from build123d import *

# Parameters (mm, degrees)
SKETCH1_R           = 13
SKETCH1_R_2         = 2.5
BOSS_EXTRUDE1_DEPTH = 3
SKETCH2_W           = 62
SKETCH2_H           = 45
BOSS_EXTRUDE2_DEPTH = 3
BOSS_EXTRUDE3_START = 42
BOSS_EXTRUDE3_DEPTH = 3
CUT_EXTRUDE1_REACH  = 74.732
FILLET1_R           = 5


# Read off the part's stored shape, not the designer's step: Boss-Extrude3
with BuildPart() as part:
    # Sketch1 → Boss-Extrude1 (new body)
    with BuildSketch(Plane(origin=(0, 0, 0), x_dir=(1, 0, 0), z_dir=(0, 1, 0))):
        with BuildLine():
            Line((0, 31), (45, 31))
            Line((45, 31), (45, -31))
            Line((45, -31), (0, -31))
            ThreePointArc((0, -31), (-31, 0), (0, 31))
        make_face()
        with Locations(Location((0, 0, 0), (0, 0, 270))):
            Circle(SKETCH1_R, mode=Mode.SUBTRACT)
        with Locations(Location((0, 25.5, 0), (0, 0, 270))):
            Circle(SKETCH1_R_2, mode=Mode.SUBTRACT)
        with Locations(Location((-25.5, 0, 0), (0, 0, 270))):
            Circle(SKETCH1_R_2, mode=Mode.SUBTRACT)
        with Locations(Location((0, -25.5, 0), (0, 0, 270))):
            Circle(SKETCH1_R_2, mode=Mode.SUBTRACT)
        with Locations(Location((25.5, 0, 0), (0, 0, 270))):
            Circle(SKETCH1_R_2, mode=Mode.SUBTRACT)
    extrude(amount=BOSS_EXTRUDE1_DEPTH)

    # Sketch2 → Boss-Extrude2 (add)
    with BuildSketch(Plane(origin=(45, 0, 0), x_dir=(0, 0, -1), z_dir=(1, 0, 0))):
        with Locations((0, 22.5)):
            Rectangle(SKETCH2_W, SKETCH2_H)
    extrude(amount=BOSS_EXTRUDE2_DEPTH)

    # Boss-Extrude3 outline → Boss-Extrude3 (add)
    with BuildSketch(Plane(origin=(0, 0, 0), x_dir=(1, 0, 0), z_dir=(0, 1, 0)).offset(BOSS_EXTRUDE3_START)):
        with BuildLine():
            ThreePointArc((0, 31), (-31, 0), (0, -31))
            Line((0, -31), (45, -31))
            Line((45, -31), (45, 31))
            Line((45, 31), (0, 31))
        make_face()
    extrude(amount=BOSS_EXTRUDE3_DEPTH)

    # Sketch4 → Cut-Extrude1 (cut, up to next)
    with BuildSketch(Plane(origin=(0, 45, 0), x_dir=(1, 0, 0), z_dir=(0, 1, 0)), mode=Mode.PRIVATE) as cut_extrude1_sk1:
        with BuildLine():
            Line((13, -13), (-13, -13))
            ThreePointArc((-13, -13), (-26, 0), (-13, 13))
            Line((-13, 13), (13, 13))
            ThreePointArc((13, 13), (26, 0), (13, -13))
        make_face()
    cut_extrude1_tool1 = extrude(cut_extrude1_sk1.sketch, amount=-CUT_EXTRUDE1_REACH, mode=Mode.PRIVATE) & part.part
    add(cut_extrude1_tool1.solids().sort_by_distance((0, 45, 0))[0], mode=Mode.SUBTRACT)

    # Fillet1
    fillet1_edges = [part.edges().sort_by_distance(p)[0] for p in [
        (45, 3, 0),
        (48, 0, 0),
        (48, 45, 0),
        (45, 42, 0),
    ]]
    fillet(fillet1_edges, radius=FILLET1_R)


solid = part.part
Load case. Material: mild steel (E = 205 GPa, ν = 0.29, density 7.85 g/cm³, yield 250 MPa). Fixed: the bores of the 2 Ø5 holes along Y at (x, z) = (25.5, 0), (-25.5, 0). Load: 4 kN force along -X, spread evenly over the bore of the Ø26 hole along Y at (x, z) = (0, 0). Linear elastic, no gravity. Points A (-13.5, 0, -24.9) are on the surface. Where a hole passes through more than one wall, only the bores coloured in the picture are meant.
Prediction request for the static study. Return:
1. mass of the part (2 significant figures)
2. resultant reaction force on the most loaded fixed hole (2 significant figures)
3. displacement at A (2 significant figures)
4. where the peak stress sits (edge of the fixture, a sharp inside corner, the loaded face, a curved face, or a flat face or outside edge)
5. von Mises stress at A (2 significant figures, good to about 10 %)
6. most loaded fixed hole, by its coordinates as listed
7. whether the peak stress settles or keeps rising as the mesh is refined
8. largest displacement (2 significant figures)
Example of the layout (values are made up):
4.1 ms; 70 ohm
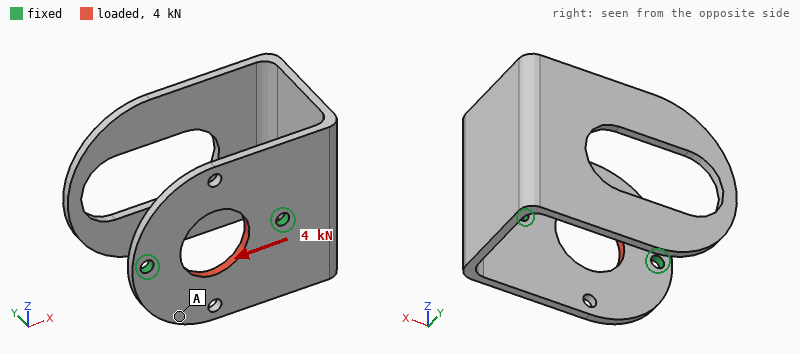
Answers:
230 g; 2.2 kN; 3.2 µm; edge of the fixture; 6.1 MPa; (25.5, 0); keeps rising; 4.2 µm
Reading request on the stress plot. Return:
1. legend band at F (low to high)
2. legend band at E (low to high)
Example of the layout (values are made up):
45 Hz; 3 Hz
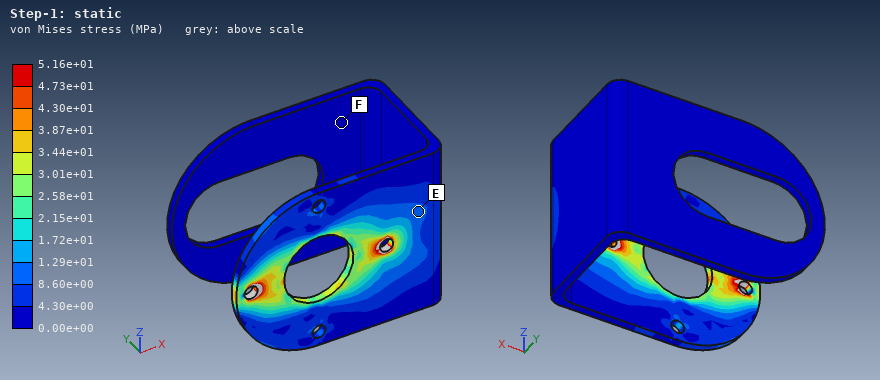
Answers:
0.00e+00 to 4.30e+00 MPa; 8.60e+00 to 1.29e+01 MPa
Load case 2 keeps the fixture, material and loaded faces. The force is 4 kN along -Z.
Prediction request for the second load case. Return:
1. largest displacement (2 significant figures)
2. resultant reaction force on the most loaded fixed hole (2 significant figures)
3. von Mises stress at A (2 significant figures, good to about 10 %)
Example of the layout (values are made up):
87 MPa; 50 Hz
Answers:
5.4 µm; 2.0 kN; 18 MPa
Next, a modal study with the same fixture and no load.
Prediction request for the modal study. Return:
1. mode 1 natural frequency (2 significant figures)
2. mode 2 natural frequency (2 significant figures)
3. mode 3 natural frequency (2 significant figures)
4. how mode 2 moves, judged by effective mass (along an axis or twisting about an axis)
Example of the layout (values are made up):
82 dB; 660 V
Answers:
260 Hz; 380 Hz; 630 Hz; along Z
